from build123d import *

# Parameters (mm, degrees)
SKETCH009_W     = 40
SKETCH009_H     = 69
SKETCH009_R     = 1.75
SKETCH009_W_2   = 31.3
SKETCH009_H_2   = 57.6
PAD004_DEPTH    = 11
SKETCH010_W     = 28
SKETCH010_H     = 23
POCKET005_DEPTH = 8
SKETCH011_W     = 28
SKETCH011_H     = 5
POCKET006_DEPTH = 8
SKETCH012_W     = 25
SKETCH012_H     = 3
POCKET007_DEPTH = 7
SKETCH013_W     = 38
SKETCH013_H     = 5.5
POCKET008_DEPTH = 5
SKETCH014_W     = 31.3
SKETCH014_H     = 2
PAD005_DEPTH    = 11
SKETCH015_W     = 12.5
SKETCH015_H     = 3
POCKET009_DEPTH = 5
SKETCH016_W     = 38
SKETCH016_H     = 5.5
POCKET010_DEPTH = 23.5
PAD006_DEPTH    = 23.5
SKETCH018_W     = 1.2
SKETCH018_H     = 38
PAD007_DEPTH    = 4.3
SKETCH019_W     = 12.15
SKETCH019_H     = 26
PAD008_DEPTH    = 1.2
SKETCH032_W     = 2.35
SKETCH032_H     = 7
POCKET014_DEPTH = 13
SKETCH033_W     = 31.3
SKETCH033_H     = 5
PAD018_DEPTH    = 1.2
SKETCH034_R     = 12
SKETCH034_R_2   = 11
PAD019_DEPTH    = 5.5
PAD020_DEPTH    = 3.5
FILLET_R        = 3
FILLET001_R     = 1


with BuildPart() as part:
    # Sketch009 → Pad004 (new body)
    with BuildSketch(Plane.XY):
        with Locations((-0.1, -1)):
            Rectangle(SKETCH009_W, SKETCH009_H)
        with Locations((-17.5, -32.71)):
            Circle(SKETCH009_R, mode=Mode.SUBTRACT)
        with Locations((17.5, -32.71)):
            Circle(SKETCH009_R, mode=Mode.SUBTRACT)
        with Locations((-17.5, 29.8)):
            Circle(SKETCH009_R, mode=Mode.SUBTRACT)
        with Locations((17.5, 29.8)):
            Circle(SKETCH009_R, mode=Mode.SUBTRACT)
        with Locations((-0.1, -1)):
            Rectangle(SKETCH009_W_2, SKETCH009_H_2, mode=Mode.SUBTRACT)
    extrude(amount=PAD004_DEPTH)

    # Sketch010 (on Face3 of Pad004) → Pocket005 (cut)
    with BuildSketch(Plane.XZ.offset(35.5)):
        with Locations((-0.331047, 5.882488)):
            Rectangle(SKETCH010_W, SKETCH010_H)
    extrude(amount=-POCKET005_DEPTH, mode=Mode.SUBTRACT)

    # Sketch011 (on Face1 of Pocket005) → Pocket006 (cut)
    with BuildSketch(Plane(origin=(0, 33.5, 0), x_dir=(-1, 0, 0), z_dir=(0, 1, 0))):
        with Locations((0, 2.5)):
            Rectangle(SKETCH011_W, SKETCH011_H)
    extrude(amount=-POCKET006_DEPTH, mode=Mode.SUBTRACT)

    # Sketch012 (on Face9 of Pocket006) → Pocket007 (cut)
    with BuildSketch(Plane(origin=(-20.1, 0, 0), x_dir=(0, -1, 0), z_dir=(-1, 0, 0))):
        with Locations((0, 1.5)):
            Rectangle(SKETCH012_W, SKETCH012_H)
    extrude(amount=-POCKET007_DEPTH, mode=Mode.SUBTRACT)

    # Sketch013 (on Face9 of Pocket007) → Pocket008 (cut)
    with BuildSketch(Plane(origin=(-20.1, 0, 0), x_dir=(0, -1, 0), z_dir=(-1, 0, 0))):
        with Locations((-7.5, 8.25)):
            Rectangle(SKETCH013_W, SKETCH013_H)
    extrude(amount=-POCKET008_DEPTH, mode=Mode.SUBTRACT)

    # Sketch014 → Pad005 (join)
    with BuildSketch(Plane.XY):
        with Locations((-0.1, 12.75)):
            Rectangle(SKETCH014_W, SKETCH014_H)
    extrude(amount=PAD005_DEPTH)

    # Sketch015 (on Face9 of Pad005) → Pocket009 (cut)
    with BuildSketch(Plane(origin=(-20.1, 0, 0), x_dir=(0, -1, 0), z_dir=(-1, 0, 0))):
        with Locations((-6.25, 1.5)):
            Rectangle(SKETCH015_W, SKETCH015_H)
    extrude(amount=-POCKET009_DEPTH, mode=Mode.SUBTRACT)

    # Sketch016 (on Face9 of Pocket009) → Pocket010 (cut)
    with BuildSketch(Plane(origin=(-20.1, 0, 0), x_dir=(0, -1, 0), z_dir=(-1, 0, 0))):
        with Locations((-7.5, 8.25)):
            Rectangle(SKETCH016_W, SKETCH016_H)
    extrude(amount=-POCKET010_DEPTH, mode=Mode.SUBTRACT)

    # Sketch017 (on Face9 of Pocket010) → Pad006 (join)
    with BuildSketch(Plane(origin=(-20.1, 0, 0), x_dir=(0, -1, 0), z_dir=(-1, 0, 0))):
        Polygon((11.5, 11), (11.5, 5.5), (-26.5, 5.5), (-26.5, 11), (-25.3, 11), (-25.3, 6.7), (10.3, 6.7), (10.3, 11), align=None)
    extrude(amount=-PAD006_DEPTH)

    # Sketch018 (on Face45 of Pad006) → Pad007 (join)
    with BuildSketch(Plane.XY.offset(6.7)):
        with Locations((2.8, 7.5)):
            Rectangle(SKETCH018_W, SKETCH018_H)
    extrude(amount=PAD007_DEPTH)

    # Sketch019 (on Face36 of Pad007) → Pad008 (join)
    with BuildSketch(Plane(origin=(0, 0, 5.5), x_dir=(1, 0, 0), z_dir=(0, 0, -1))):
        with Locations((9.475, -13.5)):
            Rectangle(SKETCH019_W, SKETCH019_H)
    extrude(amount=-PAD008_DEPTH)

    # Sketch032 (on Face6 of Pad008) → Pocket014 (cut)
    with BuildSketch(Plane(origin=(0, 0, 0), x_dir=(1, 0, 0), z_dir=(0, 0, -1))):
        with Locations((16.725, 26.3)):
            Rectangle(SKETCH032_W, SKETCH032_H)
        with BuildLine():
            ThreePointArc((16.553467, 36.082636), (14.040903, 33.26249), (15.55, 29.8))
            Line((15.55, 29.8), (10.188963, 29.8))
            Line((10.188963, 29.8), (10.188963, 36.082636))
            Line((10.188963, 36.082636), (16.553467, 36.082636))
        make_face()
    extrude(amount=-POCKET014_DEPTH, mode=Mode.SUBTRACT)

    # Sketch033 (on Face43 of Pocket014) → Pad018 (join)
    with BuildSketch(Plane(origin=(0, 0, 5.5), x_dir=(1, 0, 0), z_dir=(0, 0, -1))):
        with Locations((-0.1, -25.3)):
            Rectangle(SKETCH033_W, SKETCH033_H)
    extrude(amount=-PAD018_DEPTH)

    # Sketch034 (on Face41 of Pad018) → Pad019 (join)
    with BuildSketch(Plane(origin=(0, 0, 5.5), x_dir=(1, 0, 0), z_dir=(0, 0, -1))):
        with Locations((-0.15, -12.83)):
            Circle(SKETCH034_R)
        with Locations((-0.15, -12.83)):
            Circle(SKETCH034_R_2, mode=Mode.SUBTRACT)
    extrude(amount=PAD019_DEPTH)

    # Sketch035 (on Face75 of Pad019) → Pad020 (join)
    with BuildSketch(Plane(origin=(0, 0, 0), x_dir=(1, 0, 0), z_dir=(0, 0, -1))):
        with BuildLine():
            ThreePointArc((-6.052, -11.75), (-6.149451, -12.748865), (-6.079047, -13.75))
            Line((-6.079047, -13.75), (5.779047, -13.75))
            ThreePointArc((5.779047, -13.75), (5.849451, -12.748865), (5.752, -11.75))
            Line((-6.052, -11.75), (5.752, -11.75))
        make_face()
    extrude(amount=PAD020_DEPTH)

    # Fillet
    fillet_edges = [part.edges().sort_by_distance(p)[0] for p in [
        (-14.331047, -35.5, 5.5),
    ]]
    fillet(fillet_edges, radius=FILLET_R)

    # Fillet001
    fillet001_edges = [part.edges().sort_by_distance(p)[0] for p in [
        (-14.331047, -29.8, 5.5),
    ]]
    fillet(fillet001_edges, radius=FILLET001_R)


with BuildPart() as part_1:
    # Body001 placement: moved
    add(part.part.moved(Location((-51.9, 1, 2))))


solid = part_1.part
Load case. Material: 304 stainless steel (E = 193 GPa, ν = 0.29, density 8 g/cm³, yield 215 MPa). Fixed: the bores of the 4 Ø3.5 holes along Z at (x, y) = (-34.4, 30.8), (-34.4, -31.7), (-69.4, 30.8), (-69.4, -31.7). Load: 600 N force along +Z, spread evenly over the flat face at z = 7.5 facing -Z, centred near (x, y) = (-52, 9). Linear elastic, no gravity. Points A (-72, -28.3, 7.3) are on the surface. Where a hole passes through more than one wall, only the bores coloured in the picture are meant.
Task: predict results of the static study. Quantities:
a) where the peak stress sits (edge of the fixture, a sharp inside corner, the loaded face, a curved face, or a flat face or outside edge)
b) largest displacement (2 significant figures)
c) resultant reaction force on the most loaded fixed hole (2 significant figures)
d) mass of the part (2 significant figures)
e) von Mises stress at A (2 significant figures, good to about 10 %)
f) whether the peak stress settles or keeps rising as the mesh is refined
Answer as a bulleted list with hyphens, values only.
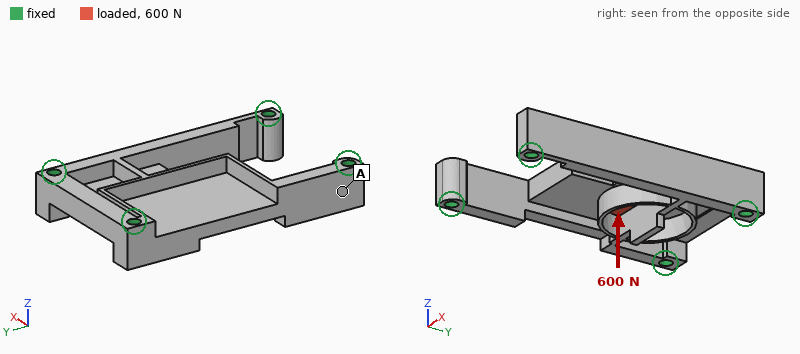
- a sharp inside corner
- 37 µm
- 230 N
- 71 g
- 12 MPa
- keeps rising
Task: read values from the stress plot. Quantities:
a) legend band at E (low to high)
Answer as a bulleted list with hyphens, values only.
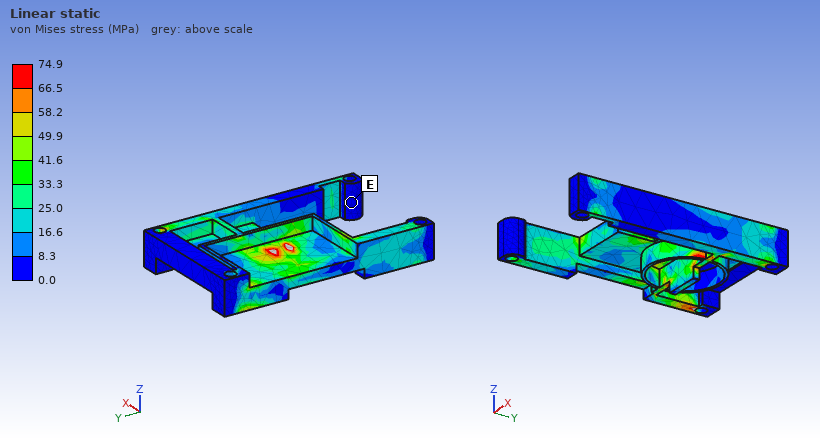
- 0.0 to 8.3 MPa
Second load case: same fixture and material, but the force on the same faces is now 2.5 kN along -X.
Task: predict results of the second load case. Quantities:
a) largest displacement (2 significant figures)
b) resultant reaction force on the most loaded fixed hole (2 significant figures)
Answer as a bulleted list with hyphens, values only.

- 19 µm
- 1.7 kN
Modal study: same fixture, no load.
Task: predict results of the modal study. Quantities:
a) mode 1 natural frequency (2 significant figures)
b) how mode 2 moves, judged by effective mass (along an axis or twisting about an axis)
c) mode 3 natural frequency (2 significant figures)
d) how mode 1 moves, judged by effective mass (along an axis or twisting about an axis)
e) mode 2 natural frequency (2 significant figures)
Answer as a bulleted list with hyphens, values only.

- 6300 Hz
- along X
- 11 kHz
- along Z
- 9700 Hz
